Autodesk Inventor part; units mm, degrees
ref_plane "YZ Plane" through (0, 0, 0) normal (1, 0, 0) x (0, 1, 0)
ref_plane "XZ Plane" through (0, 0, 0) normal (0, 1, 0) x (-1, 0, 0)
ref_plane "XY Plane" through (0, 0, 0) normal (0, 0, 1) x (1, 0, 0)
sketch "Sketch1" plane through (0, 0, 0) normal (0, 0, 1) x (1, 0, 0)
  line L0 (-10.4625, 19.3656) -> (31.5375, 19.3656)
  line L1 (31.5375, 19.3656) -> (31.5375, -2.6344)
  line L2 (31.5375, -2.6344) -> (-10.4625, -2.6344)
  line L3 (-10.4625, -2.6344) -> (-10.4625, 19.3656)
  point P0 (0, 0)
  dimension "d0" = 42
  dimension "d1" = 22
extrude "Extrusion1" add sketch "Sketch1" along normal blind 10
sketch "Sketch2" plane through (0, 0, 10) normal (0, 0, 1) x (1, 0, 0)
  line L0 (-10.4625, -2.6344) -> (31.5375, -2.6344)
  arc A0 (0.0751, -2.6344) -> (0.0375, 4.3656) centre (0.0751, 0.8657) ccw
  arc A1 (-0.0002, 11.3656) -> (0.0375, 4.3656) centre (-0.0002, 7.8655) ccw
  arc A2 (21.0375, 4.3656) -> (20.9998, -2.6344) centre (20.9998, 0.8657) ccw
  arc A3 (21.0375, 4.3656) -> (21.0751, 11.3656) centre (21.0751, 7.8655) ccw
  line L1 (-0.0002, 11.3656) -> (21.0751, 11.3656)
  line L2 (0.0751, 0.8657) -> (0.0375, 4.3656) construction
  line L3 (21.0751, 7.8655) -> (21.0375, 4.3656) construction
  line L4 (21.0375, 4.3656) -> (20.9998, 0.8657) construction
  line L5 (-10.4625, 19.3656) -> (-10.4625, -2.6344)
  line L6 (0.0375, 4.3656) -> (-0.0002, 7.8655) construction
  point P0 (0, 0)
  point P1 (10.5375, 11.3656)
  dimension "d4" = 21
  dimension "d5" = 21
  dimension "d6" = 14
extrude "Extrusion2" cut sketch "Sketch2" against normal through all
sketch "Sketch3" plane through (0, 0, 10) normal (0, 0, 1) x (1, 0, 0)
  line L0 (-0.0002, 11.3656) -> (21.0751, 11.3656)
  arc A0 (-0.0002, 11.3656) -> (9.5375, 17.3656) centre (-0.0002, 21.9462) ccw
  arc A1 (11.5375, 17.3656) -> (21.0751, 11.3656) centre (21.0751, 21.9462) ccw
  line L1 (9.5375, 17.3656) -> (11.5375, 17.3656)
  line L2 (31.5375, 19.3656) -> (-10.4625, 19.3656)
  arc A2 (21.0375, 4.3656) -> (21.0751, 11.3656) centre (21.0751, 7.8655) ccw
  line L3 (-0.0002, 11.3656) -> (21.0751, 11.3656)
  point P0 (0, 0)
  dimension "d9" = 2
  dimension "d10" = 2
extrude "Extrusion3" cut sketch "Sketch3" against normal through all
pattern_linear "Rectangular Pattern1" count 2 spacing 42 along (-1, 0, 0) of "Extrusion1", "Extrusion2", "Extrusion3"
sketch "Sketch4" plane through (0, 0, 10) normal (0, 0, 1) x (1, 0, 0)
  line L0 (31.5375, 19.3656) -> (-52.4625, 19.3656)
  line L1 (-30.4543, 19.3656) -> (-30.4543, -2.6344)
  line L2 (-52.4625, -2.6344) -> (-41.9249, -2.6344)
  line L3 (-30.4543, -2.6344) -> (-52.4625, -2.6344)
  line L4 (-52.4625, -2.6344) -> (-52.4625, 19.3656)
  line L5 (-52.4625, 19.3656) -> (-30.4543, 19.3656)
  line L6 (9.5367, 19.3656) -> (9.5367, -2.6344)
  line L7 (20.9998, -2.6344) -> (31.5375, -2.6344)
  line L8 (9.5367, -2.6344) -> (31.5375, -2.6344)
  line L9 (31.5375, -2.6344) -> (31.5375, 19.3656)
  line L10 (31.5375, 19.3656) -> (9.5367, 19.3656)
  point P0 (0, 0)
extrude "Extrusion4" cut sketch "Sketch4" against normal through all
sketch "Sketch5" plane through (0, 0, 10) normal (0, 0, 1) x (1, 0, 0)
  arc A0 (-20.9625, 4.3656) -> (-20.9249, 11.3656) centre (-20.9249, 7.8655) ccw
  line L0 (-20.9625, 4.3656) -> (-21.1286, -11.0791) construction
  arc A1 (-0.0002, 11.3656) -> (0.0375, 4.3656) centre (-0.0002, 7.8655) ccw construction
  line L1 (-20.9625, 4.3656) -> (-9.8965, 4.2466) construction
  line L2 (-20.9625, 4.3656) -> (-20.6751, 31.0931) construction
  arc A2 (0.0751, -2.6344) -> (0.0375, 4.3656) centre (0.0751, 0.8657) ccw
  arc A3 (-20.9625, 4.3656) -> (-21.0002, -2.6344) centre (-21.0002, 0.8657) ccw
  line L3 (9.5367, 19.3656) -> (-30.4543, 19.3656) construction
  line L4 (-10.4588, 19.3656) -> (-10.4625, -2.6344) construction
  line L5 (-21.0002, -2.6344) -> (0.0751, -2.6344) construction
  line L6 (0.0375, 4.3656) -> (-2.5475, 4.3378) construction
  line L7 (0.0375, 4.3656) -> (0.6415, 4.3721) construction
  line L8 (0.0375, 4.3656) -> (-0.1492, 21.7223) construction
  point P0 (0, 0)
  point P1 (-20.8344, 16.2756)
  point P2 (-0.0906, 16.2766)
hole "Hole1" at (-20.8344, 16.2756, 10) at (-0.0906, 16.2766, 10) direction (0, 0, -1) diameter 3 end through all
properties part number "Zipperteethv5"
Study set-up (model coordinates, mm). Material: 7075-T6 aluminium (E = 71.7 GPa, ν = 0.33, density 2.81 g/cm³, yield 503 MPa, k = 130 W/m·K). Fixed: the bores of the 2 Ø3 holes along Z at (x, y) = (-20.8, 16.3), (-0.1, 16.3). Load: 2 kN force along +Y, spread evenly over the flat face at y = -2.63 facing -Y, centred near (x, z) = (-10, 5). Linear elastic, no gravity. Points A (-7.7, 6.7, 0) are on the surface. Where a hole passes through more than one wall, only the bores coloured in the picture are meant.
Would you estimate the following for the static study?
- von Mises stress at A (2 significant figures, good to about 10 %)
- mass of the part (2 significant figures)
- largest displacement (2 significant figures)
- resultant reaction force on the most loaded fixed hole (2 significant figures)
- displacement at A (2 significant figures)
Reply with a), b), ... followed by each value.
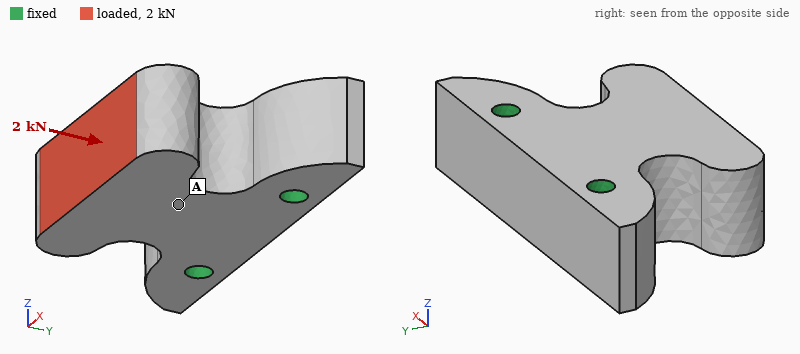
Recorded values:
a) 9.5 MPa
b) 16 g
c) 6.0 µm
d) 1.1 kN
e) 3.4 µm
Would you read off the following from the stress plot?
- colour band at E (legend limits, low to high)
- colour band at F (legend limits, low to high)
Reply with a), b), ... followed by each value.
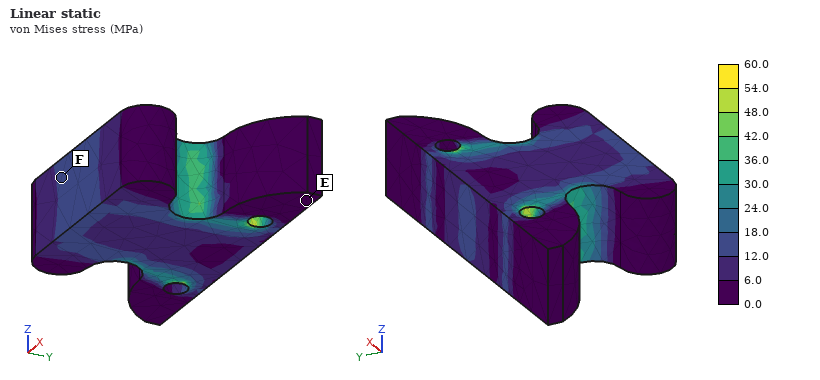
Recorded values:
a) 0.0 to 6.0 MPa
b) 12.0 to 18.0 MPa
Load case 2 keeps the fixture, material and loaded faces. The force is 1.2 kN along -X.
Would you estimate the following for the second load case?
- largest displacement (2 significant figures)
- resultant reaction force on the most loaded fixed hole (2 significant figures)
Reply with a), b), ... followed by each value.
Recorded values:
a) 19 µm
b) 1.3 kN
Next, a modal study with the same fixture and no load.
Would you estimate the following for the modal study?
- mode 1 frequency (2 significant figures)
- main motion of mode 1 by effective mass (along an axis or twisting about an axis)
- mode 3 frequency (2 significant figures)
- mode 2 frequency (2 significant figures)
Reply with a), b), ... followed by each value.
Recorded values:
a) 12 kHz
b) along Z
c) 21 kHz
d) 21 kHz
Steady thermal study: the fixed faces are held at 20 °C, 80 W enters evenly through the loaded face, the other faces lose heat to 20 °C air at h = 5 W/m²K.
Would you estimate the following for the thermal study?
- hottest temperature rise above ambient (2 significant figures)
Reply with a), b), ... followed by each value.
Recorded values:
a) 76 K
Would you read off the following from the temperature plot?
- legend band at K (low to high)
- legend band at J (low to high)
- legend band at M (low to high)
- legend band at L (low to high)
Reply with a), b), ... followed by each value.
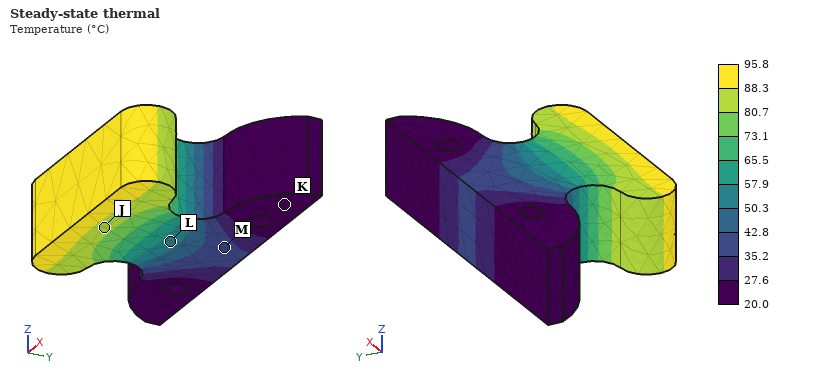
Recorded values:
a) 20.0 to 27.6 °C
b) 80.7 to 88.3 °C
c) 35.2 to 42.8 °C
d) 50.3 to 57.9 °C
